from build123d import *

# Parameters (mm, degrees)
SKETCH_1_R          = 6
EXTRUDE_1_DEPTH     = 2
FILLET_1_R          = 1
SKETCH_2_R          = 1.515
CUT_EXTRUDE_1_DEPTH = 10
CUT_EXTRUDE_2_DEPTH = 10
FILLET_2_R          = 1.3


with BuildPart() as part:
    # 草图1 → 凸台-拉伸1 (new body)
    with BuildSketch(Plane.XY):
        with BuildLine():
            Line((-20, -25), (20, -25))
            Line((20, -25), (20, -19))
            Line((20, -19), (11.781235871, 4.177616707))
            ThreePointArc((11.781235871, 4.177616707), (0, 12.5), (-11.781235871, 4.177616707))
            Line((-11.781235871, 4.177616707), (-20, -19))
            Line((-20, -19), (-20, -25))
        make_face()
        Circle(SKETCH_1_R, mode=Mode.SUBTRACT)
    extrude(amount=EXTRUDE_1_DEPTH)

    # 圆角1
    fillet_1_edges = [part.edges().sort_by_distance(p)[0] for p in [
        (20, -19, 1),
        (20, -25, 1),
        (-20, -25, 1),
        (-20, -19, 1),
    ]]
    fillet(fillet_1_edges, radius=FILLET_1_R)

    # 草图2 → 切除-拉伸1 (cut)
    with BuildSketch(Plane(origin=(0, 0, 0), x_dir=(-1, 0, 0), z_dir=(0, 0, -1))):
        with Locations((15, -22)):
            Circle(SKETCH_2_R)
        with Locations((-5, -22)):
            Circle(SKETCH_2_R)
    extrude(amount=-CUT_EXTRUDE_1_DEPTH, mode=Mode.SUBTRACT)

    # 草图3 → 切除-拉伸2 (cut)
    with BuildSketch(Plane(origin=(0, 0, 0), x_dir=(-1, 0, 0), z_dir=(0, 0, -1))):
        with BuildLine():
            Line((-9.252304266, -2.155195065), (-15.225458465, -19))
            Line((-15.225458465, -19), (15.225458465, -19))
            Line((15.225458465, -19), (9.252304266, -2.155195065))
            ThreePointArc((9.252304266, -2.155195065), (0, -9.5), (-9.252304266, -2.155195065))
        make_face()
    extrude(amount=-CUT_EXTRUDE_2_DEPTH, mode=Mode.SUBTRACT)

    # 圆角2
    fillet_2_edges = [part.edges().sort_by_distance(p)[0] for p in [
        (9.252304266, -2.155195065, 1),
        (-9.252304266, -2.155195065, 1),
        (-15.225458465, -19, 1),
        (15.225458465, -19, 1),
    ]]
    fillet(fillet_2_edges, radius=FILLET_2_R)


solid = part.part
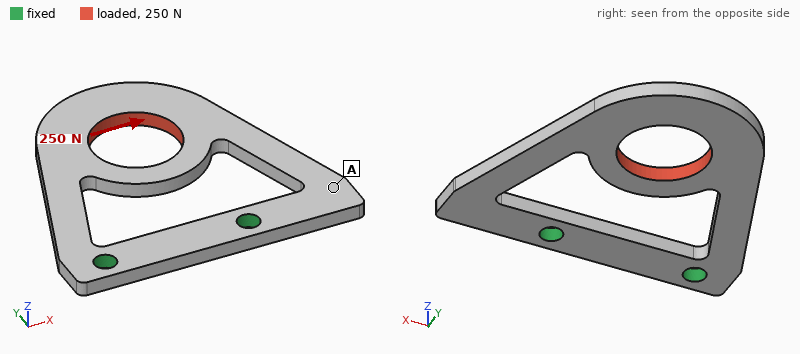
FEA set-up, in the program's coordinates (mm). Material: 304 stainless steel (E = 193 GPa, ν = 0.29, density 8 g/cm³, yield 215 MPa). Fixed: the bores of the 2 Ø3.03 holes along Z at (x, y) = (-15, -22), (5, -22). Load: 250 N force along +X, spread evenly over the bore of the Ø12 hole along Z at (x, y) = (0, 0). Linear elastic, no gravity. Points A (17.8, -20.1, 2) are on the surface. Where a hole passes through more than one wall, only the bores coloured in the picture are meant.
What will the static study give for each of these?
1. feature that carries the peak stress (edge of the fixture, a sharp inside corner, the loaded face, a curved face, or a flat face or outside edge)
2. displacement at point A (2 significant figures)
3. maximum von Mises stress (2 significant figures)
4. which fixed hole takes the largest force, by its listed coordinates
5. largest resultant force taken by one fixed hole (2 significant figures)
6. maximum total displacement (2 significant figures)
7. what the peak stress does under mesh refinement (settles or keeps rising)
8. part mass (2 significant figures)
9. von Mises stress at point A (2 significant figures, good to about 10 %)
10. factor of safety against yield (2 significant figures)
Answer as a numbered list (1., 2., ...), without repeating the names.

1. a curved face
2. 18 µm
3. 230 MPa
4. (-15, -22)
5. 200 N
6. 39 µm
7. settles
8. 11 g
9. 21 MPa
10. 0.92
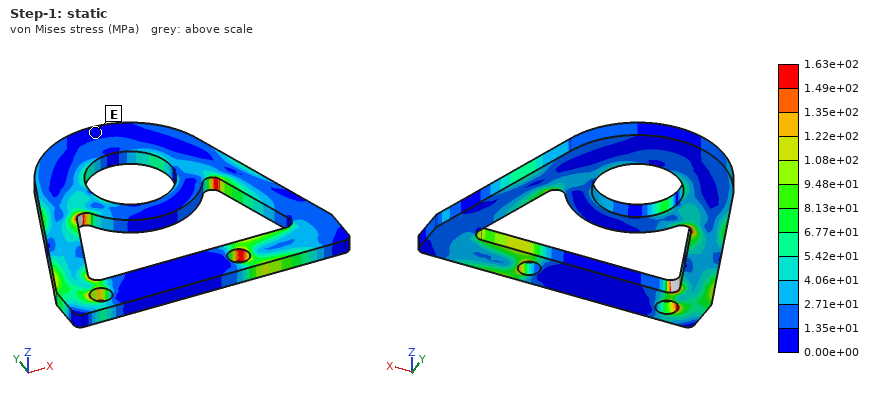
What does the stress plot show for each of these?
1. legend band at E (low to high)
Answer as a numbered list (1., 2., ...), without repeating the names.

1. 0.00e+00 to 1.35e+01 MPa
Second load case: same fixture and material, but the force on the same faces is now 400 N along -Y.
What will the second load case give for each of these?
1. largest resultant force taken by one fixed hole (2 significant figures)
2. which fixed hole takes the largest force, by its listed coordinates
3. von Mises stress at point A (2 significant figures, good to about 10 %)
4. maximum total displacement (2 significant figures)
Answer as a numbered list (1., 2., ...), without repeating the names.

1. 220 N
2. (5, -22)
3. 14 MPa
4. 23 µm
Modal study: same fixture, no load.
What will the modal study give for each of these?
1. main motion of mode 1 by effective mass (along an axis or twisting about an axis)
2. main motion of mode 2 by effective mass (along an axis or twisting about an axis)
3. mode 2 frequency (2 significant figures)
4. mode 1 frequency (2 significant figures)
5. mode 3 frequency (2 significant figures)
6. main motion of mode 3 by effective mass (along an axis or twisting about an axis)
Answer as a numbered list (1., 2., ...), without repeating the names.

1. along Z
2. twisting about Y
3. 3300 Hz
4. 950 Hz
5. 5100 Hz
6. along X
